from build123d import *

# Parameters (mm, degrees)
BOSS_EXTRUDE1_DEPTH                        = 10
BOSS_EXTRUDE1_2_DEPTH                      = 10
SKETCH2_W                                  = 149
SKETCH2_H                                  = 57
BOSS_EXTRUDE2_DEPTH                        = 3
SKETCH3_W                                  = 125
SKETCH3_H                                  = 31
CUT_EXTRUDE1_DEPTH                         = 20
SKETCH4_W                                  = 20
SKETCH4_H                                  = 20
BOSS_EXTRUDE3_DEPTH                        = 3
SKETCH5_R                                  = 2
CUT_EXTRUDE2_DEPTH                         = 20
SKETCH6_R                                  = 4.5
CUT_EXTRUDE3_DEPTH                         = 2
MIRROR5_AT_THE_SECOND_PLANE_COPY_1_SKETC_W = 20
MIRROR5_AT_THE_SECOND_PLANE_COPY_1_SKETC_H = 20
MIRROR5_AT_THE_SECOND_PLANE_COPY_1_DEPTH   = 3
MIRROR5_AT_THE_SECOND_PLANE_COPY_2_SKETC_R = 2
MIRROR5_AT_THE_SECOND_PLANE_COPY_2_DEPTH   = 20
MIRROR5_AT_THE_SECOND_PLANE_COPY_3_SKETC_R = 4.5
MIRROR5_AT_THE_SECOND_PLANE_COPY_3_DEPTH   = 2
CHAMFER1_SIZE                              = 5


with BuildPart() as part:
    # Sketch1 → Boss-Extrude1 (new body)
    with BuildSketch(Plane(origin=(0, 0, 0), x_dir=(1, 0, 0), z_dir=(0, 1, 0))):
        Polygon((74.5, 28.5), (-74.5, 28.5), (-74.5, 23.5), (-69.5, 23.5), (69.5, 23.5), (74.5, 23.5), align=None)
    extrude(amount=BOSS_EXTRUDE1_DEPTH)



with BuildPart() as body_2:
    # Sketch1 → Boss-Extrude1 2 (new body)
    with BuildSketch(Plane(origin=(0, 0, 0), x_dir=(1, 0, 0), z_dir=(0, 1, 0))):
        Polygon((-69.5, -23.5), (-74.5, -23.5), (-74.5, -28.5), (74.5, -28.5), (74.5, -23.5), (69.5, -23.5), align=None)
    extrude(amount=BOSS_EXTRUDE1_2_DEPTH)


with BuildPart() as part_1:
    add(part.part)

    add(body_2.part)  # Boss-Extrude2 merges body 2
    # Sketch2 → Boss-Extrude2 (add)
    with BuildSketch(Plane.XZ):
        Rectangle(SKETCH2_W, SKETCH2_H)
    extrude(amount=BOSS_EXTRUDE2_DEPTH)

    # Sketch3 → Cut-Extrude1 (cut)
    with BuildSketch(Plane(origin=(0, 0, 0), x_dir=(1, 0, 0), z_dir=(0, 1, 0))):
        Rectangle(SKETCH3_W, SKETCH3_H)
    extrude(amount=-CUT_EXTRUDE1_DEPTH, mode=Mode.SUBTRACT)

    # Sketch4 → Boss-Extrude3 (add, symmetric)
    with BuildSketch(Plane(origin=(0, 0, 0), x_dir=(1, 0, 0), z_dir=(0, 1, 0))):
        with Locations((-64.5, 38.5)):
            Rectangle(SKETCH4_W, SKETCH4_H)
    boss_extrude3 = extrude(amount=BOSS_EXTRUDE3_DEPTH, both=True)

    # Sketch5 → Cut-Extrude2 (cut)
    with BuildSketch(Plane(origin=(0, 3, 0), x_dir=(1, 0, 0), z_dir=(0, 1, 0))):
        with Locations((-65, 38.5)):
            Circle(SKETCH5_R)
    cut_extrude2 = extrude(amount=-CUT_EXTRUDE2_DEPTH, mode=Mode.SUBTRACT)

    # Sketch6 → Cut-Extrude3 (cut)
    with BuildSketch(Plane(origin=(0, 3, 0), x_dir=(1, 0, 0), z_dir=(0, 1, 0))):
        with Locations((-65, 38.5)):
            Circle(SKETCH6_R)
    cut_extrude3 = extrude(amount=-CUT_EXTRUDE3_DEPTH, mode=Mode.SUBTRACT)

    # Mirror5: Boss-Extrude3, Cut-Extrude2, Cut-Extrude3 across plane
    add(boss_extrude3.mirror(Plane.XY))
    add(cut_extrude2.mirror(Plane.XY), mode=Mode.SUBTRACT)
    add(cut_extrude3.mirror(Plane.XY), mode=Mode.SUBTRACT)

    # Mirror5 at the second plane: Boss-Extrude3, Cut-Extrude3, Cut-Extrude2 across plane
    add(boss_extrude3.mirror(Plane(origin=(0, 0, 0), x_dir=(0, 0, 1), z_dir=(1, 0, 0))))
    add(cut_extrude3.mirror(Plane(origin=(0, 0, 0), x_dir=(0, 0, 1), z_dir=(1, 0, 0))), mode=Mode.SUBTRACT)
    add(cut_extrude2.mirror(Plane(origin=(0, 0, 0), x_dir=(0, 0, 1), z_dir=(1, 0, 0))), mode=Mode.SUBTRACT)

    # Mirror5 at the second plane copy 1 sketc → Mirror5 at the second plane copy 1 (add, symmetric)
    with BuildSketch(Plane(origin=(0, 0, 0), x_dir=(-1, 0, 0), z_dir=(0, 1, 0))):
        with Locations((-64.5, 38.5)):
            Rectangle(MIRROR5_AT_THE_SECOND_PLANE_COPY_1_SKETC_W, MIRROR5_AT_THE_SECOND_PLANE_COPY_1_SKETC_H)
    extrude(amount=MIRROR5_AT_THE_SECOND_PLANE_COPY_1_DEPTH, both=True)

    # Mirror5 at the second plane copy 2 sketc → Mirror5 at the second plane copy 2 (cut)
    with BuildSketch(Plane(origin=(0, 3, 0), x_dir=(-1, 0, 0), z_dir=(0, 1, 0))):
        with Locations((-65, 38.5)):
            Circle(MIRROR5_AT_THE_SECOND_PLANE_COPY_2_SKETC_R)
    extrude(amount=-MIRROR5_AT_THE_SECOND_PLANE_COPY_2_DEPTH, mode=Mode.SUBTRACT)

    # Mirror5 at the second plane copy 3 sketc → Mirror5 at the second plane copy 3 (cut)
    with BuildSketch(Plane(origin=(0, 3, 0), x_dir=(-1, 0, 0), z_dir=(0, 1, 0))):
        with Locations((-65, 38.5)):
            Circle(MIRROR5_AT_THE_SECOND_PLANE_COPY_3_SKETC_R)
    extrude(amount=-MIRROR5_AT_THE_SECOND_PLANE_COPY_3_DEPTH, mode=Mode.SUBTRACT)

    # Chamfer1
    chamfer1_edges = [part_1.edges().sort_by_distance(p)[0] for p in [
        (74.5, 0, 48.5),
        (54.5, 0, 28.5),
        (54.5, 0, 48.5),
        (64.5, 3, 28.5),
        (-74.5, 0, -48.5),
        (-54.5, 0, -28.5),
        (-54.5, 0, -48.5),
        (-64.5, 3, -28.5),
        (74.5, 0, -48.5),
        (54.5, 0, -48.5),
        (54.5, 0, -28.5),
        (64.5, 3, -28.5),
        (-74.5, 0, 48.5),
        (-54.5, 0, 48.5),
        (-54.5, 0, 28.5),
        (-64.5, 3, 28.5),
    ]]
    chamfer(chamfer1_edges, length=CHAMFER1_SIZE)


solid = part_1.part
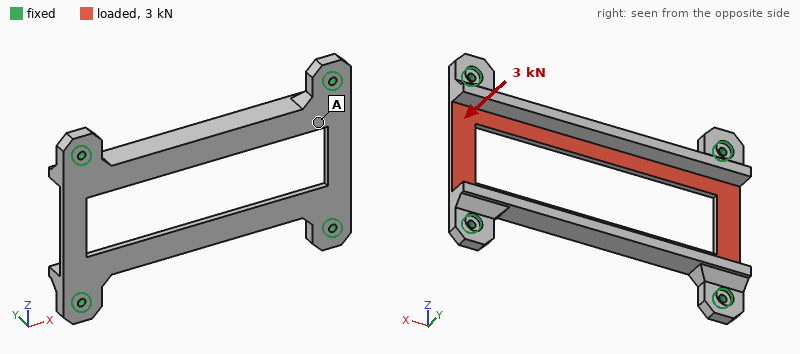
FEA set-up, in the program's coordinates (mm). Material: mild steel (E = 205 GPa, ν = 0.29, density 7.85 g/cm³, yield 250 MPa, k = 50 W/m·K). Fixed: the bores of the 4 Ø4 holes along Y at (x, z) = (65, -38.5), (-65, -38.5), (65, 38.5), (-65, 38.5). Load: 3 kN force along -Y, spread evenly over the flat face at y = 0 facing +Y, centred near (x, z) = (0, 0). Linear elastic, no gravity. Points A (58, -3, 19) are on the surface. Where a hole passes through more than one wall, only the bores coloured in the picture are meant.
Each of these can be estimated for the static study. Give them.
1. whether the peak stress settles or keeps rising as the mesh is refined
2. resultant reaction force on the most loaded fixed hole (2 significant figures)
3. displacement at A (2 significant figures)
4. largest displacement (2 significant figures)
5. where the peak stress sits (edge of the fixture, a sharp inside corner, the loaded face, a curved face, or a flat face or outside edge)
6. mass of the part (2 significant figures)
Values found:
keeps rising
950 N
0.051 mm
0.12 mm
edge of the fixture
300 g
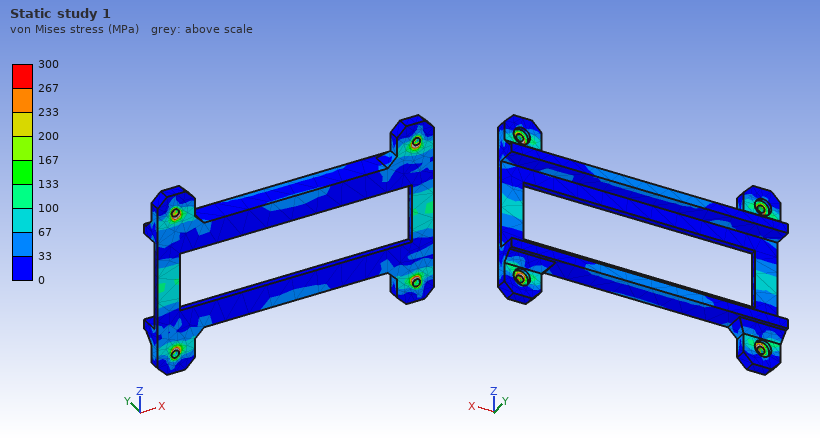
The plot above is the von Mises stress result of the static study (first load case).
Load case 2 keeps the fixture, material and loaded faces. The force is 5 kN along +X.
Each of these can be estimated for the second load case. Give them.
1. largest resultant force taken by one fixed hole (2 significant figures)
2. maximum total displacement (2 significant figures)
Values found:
1.3 kN
24 µm
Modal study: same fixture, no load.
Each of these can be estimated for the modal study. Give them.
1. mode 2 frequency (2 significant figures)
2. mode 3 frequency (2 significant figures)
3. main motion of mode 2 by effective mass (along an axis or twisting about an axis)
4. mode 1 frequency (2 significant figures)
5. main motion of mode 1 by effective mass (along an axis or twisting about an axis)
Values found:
2300 Hz
3400 Hz
twisting about X
2200 Hz
along Y
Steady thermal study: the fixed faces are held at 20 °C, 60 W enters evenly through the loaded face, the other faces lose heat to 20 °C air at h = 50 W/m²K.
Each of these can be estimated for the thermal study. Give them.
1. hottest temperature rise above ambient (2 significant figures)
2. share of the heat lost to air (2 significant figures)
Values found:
51 K
43 %
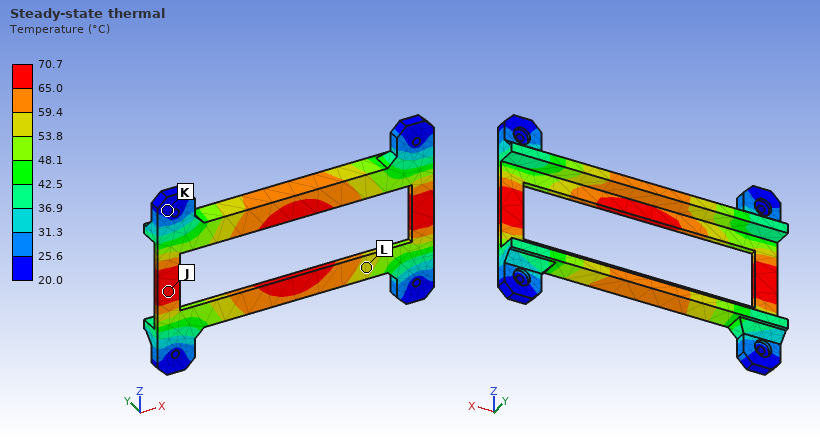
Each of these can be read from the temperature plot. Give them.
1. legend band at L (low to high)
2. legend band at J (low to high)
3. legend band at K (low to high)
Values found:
53.8 to 59.4 °C
65.0 to 70.7 °C
20.0 to 25.6 °C
